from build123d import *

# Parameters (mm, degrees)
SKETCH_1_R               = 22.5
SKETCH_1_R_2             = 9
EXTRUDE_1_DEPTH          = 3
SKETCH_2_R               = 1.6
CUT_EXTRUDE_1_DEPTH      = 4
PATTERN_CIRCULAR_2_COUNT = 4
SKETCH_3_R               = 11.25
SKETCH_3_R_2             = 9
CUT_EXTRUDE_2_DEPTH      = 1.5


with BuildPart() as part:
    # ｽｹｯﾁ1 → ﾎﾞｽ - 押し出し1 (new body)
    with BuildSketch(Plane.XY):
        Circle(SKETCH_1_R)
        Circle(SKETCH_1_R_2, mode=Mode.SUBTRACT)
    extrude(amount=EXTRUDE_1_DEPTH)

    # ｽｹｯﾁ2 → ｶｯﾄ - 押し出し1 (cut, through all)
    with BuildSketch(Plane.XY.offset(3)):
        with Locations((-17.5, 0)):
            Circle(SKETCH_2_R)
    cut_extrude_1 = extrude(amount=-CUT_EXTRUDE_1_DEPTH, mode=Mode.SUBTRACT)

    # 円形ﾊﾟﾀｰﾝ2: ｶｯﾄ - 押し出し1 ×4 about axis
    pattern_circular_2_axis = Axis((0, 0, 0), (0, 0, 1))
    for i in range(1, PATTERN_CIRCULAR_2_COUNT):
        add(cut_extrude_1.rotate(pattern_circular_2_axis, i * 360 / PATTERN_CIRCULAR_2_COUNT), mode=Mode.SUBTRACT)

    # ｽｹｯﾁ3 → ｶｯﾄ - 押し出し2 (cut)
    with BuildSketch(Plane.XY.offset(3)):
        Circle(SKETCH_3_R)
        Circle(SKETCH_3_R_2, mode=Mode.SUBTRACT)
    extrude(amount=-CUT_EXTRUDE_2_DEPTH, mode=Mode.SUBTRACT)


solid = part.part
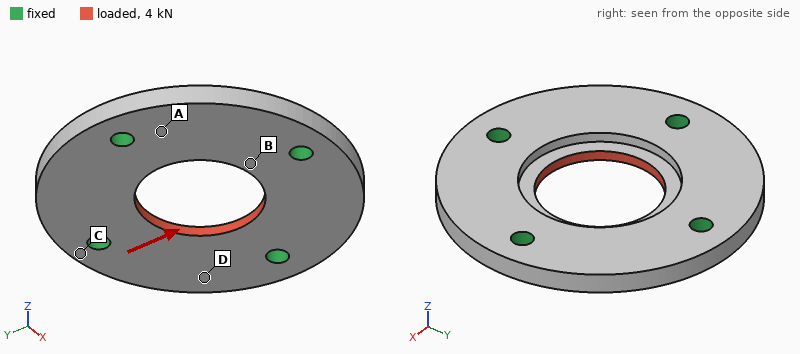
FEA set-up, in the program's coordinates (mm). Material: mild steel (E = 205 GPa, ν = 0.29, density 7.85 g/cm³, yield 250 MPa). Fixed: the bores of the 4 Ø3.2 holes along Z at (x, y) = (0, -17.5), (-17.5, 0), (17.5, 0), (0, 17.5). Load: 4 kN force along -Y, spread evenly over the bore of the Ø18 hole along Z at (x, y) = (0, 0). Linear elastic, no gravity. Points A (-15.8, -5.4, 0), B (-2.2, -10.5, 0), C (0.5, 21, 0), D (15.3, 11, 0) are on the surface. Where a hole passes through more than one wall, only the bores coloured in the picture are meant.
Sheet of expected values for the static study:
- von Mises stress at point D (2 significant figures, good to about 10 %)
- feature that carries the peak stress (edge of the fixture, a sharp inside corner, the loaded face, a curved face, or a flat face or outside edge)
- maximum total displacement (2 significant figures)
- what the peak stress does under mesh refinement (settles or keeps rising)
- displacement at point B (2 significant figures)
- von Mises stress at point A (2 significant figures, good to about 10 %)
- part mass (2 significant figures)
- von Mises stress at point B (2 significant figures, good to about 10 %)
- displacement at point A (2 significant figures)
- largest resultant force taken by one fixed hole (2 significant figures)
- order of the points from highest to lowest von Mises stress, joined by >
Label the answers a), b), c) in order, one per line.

a) 14 MPa
b) edge of the fixture
c) 3.8 µm
d) keeps rising
e) 2.6 µm
f) 26 MPa
g) 29 g
h) 64 MPa
i) 1.1 µm
j) 1.1 kN
k) B > A > D > C
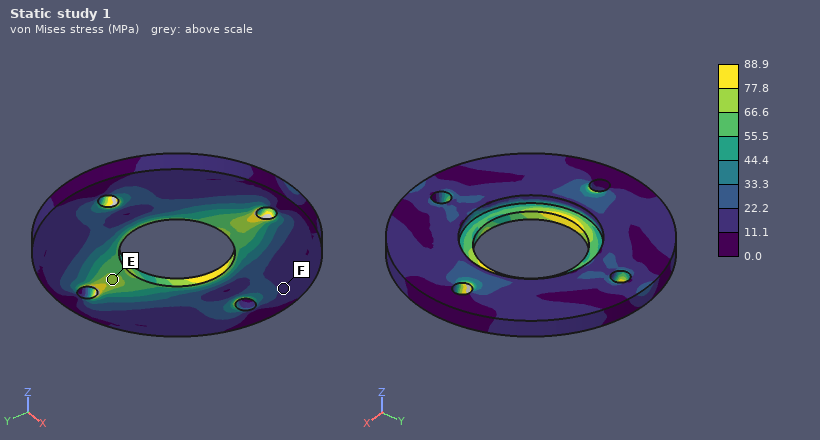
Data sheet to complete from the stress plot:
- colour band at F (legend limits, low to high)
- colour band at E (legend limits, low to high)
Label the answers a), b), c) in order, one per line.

a) 11.1 to 22.2 MPa
b) 66.6 to 77.8 MPa
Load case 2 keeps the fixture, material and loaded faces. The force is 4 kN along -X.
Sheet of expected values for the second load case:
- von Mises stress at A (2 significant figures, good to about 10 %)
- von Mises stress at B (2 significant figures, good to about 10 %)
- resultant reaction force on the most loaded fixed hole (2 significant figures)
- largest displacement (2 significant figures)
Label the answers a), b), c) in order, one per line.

a) 30 MPa
b) 33 MPa
c) 1.1 kN
d) 3.8 µm
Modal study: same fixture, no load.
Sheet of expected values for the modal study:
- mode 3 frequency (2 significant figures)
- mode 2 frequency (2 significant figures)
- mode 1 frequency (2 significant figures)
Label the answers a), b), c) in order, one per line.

a) 18 kHz
b) 18 kHz
c) 18 kHz
